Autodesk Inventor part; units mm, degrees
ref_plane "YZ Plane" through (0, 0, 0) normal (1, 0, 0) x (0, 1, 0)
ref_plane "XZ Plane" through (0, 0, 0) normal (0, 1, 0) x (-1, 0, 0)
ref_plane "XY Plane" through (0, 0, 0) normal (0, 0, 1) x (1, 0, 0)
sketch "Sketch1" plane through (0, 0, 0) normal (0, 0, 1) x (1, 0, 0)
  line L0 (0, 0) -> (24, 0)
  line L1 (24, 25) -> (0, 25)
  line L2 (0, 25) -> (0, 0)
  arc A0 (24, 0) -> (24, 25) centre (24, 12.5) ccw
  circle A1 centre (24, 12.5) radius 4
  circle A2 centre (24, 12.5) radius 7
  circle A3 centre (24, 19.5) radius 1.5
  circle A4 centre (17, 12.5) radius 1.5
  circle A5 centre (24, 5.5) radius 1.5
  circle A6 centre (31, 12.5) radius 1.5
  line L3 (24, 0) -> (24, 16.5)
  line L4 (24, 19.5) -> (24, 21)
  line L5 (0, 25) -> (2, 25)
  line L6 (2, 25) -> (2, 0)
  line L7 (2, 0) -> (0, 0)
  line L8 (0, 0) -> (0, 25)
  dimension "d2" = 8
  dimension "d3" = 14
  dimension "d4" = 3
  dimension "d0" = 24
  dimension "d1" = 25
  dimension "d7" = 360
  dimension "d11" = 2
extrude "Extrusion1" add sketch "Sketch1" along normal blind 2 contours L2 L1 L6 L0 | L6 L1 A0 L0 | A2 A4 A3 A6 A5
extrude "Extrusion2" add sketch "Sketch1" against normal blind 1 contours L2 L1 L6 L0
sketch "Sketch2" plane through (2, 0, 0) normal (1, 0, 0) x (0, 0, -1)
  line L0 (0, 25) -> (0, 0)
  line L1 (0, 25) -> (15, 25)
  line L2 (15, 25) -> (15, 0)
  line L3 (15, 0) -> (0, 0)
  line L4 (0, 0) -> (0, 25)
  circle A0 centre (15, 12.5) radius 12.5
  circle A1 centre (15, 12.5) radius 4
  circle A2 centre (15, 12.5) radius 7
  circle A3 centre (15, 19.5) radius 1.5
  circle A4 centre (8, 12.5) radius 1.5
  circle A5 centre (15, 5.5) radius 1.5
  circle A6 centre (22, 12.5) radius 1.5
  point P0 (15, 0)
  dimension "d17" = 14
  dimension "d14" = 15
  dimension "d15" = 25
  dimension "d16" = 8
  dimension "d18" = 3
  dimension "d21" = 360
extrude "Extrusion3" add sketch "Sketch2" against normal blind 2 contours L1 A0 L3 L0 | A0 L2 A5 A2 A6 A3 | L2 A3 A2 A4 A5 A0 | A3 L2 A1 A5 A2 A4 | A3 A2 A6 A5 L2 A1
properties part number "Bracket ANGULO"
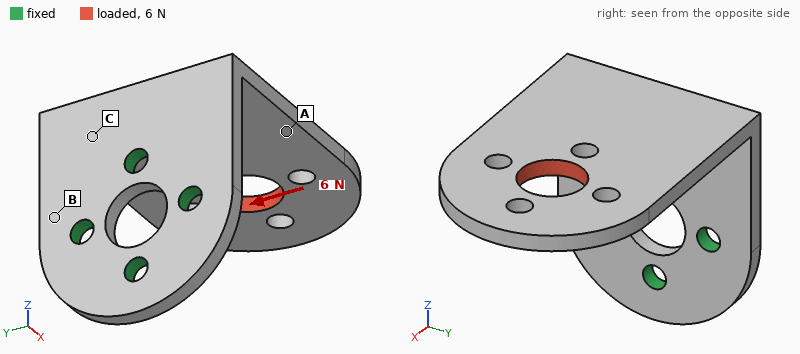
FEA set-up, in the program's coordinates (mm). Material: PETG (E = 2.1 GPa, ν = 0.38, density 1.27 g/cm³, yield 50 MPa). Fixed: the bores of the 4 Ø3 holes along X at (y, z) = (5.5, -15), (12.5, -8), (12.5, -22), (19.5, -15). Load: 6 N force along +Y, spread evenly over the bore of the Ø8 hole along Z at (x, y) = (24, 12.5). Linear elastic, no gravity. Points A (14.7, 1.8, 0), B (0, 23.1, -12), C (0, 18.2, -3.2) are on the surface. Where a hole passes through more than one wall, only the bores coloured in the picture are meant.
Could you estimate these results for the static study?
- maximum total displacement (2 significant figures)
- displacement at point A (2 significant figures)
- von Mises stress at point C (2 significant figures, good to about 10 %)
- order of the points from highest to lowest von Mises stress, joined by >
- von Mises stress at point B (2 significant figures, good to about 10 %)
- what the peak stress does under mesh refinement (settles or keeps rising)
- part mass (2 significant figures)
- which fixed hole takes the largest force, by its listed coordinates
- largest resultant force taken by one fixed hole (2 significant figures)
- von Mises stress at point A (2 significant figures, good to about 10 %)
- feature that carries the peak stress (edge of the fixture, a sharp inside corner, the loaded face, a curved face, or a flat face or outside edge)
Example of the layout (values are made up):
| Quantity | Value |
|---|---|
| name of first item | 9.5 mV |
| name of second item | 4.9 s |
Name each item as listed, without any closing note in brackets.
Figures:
| Quantity | Value |
|---|---|
| maximum total displacement | 0.62 mm |
| displacement at point A | 0.31 mm |
| von Mises stress at point C | 2.9 MPa |
| order of the points from highest to lowest von Mises stress, joined by > | B > C > A |
| von Mises stress at point B | 4.2 MPa |
| what the peak stress does under mesh refinement | keeps rising |
| part mass | 3.3 g |
| which fixed hole takes the largest force, by its listed coordinates | (12.5, -8) |
| largest resultant force taken by one fixed hole | 6.1 N |
| von Mises stress at point A | 0.82 MPa |
| feature that carries the peak stress | edge of the fixture |
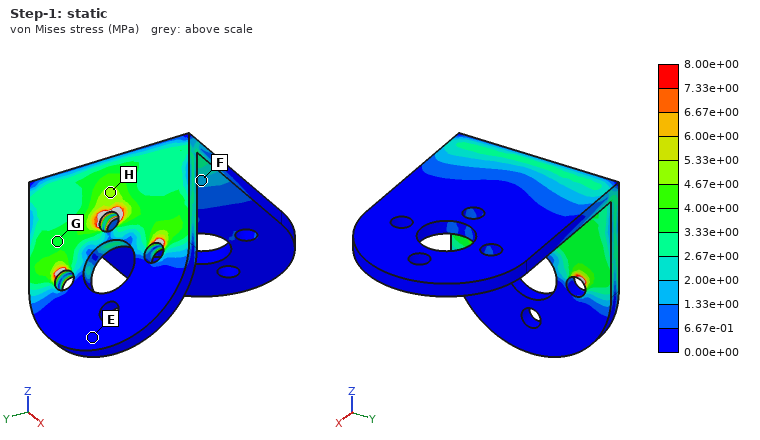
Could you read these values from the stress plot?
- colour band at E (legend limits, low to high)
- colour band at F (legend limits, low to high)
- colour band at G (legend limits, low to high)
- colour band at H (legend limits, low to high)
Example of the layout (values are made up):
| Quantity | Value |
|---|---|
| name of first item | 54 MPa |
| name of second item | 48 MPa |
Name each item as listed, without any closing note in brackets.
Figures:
| Quantity | Value |
|---|---|
| colour band at E | 0.00e+00 to 6.67e-01 MPa |
| colour band at F | 1.33e+00 to 2.00e+00 MPa |
| colour band at G | 3.33e+00 to 4.00e+00 MPa |
| colour band at H | 4.67e+00 to 5.33e+00 MPa |
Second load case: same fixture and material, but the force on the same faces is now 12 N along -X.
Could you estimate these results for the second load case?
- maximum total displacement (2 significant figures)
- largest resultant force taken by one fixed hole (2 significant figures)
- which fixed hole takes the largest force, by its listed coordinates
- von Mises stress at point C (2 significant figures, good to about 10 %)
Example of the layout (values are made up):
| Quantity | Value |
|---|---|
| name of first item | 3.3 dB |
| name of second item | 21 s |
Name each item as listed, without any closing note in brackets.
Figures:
| Quantity | Value |
|---|---|
| maximum total displacement | 0.51 mm |
| largest resultant force taken by one fixed hole | 16 N |
| which fixed hole takes the largest force, by its listed coordinates | (12.5, -8) |
| von Mises stress at point C | 2.7 MPa |
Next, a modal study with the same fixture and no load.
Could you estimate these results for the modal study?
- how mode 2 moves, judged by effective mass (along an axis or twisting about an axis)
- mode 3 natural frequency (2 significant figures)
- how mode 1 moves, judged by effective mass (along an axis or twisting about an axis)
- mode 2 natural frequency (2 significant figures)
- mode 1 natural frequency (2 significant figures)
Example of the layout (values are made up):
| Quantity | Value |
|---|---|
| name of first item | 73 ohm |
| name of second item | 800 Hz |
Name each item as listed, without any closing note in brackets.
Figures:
| Quantity | Value |
|---|---|
| how mode 2 moves, judged by effective mass | along Y |
| mode 3 natural frequency | 1100 Hz |
| how mode 1 moves, judged by effective mass | along Z |
| mode 2 natural frequency | 510 Hz |
| mode 1 natural frequency | 290 Hz |
